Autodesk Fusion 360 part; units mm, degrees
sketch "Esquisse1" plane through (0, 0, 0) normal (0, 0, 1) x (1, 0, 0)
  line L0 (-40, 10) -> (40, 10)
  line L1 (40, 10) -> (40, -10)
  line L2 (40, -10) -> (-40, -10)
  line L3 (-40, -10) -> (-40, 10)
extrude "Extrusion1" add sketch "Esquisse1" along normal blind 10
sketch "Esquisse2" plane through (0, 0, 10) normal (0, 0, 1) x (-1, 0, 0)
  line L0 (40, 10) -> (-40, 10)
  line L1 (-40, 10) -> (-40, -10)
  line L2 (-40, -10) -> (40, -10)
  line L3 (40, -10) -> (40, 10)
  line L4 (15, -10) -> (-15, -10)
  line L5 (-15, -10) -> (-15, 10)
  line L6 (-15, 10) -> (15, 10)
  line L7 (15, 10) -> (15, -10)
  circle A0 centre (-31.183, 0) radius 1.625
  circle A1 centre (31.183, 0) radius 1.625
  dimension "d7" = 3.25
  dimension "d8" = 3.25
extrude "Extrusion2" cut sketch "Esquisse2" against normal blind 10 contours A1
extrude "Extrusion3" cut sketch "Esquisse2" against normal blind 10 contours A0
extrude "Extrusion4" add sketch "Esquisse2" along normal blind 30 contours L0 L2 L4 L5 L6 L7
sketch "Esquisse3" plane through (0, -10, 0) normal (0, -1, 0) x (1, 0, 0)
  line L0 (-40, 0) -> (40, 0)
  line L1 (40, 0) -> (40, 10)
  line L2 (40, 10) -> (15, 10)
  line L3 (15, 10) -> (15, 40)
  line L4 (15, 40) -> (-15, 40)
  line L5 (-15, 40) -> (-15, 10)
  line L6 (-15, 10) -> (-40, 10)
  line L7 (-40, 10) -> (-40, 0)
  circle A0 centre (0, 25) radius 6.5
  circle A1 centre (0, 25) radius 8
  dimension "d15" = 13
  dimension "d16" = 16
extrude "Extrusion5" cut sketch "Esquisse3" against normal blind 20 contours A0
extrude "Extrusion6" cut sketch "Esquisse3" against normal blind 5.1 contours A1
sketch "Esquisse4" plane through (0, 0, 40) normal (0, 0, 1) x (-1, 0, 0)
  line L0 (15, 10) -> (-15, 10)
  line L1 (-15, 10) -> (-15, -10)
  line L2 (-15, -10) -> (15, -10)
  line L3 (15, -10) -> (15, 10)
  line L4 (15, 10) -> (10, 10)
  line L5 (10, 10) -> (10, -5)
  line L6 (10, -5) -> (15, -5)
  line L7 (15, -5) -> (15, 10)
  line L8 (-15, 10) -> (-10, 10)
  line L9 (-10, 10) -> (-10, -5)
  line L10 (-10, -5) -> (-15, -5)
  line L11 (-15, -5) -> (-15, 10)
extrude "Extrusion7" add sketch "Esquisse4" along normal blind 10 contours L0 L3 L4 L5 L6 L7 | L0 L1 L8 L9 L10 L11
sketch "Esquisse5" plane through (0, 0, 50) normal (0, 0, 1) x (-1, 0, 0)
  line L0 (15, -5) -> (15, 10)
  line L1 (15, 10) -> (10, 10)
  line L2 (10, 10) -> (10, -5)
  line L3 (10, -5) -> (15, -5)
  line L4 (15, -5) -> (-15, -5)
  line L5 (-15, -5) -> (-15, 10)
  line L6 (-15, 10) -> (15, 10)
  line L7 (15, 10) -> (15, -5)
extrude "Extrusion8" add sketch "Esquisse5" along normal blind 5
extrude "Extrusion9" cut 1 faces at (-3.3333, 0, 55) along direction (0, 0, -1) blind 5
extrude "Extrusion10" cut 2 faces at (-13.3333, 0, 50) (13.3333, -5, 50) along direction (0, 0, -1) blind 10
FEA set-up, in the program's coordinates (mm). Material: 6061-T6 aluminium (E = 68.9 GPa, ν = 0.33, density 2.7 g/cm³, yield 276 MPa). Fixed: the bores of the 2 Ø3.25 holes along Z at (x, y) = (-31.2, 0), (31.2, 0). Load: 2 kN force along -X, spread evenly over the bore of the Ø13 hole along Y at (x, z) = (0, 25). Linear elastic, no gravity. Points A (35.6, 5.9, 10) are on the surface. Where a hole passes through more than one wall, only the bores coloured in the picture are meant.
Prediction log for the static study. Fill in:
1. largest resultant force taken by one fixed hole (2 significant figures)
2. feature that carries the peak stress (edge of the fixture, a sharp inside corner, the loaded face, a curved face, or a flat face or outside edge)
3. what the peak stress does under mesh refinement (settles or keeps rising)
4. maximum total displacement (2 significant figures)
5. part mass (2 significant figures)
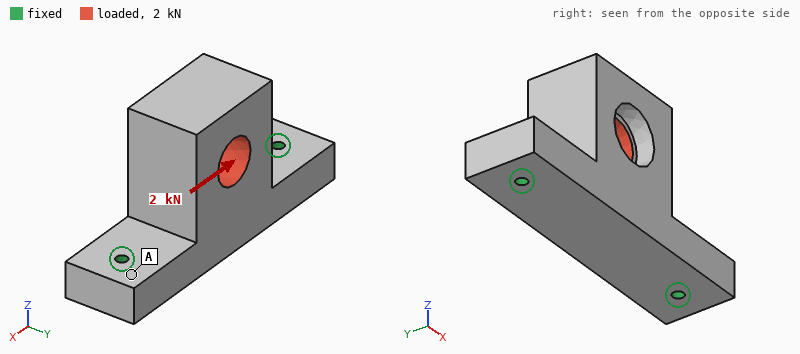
1.3 kN
edge of the fixture
keeps rising
26 µm
83 g
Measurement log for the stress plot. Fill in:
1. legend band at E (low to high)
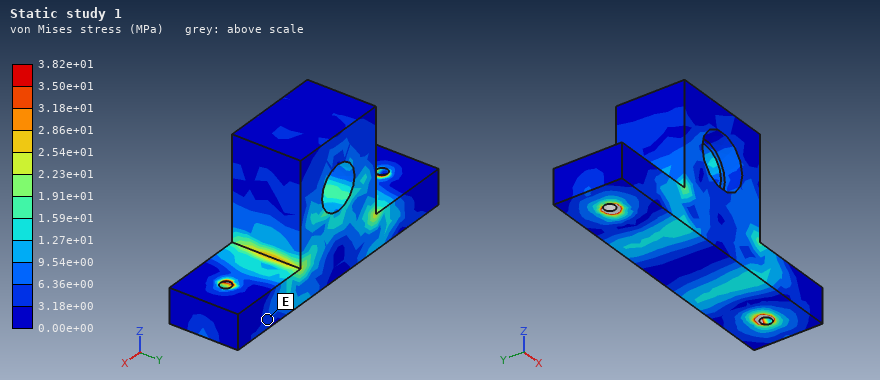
3.18e+00 to 6.36e+00 MPa
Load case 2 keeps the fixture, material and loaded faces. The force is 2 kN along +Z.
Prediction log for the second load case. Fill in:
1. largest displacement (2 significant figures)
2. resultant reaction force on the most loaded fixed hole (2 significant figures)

26 µm
1.1 kN
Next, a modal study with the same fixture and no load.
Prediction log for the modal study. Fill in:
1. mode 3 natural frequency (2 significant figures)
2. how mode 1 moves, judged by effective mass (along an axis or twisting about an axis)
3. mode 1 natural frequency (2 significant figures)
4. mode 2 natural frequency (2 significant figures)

7900 Hz
along Y
3300 Hz
7700 Hz
